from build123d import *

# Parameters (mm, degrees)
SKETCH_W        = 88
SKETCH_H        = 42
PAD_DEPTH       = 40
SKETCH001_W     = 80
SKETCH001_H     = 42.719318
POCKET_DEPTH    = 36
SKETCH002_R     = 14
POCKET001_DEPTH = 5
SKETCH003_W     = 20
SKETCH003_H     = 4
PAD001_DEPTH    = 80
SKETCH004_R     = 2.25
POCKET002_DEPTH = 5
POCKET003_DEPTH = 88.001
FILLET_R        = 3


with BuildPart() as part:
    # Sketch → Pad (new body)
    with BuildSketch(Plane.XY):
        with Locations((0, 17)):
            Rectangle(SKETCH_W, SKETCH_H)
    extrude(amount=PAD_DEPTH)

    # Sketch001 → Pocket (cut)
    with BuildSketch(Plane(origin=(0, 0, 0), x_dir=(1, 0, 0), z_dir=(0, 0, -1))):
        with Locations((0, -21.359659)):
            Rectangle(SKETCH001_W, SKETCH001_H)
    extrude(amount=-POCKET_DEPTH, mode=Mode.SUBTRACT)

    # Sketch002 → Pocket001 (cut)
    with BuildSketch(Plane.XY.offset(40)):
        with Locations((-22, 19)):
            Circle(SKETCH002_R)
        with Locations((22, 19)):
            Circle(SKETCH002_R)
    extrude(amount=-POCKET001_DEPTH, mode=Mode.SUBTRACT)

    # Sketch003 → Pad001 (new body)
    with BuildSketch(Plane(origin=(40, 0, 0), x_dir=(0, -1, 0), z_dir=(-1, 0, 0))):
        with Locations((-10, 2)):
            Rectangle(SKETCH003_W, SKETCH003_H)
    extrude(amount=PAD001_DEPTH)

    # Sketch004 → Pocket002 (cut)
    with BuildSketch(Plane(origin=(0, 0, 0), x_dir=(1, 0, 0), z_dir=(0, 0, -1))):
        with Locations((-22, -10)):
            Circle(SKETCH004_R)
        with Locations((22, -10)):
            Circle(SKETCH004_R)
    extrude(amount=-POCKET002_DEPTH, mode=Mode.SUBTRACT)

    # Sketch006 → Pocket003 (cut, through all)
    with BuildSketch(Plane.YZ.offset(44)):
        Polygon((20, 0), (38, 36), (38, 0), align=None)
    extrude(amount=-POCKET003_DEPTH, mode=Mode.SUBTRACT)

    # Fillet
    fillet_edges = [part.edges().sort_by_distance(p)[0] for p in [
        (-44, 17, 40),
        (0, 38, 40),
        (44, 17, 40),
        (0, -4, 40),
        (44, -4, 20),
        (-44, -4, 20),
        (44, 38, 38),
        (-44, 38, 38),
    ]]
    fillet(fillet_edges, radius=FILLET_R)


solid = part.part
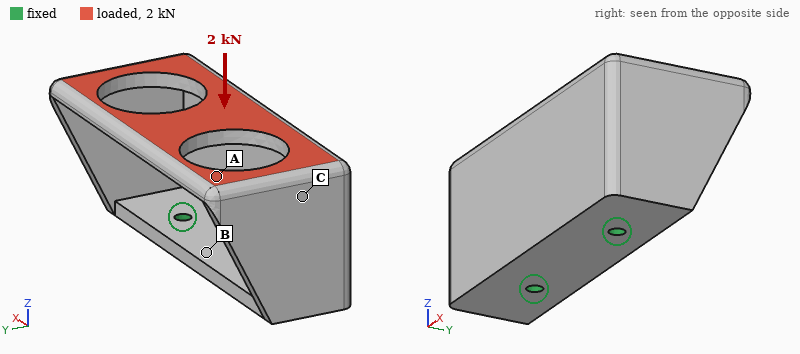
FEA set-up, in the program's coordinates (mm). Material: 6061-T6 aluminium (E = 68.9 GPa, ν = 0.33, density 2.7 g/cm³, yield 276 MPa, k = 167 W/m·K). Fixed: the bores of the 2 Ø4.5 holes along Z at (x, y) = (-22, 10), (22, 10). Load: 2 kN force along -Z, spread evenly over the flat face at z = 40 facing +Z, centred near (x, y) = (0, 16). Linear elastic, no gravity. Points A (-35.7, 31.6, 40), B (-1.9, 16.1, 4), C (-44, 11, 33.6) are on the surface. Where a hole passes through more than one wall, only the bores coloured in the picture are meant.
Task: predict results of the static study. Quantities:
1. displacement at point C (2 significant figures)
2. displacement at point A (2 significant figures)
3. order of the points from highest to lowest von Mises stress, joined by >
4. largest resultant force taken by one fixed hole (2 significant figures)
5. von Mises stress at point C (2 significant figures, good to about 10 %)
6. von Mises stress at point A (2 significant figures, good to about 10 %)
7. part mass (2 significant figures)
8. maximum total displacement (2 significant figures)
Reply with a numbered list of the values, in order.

1. 0.28 mm
2. 0.46 mm
3. A > C > B
4. 1.0 kN
5. 36 MPa
6. 68 MPa
7. 99 g
8. 0.76 mm
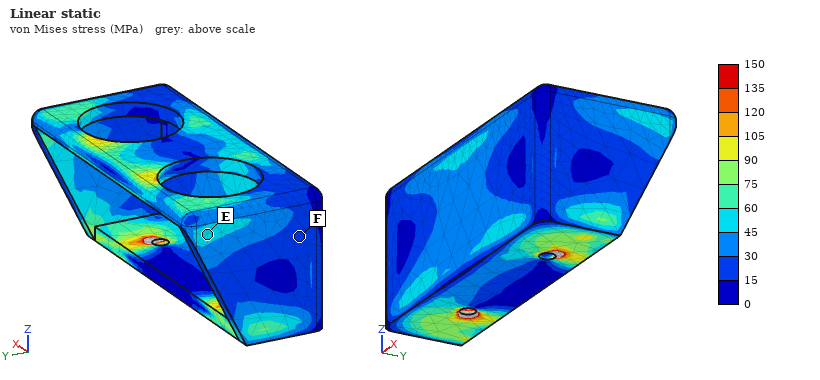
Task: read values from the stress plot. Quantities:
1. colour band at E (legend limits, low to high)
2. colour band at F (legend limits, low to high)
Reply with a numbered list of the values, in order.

1. 45 to 60 MPa
2. 15 to 30 MPa
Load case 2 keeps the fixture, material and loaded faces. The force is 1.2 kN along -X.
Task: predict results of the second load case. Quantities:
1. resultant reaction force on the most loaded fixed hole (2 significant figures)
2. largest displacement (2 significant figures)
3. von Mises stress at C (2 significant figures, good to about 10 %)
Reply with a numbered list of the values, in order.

1. 1.1 kN
2. 0.32 mm
3. 18 MPa
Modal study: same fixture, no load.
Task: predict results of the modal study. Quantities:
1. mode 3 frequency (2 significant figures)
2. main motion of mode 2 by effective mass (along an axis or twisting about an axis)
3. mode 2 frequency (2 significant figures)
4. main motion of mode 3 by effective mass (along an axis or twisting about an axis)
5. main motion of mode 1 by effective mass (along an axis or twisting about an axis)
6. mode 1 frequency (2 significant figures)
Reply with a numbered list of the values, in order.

1. 3000 Hz
2. along X
3. 1500 Hz
4. along Z
5. along Y
6. 990 Hz
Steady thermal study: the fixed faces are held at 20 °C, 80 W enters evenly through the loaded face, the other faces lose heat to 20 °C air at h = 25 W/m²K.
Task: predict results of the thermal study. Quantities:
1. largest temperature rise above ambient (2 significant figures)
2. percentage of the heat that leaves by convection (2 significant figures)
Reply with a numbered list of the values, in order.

1. 79 K
2. 19 %
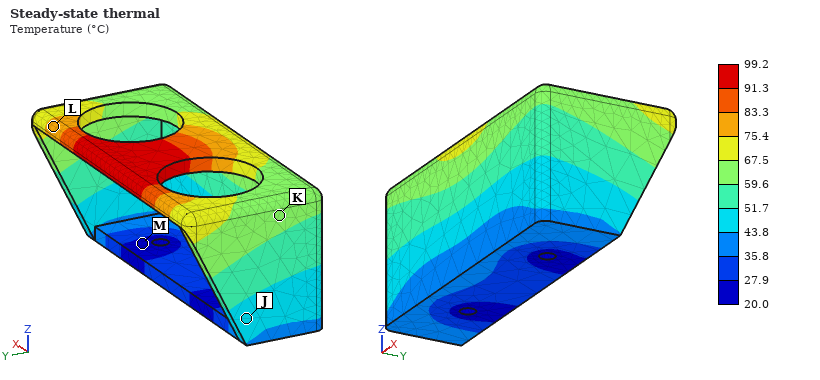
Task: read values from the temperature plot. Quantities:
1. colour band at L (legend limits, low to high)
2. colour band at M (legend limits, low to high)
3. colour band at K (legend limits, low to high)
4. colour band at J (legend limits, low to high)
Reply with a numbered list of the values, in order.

1. 75.4 to 83.3 °C
2. 20.0 to 27.9 °C
3. 59.6 to 67.5 °C
4. 43.8 to 51.7 °C
